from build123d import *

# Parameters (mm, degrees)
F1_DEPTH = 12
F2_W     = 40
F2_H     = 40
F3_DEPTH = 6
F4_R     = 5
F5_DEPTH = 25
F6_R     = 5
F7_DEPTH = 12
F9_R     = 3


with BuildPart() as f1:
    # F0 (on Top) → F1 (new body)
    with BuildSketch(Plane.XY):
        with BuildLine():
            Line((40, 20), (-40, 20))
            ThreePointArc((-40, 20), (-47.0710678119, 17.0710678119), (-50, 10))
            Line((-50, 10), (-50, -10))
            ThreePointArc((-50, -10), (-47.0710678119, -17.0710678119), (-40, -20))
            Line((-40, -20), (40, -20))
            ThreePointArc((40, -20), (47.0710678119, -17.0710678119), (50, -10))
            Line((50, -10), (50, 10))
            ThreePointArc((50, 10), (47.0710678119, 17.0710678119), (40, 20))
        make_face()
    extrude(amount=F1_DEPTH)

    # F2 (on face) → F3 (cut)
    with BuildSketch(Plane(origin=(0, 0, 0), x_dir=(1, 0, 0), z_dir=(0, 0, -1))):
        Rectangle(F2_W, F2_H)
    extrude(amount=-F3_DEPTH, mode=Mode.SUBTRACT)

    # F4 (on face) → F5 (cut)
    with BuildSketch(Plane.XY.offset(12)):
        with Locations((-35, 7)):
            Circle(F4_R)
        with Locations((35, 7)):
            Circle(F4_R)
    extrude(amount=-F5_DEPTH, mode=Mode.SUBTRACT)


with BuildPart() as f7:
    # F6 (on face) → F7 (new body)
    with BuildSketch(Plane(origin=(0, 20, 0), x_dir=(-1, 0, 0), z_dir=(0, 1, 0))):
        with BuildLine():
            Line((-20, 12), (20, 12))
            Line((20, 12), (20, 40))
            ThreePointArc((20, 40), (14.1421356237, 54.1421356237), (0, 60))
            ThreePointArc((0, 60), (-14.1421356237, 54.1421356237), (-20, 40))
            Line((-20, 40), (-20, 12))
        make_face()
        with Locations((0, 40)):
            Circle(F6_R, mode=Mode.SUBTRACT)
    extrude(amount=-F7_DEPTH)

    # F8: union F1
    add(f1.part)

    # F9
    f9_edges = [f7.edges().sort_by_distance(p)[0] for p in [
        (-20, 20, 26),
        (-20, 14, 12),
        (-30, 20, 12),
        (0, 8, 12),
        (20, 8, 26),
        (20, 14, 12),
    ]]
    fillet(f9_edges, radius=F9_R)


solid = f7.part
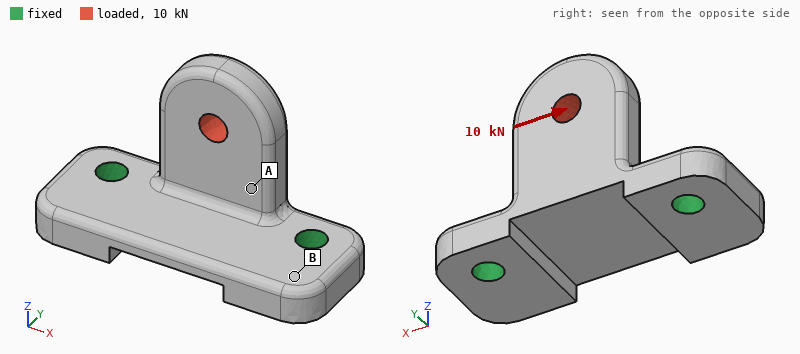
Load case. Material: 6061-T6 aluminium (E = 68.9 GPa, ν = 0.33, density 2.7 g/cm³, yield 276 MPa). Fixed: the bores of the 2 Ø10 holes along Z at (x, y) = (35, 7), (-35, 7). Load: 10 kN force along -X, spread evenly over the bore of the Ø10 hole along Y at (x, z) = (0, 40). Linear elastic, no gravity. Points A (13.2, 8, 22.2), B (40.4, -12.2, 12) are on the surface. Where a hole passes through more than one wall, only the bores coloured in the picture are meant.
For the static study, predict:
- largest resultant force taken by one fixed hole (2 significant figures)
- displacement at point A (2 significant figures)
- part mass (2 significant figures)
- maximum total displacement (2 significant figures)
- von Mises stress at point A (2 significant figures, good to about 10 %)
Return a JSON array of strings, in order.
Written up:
["8.6 kN", "0.053 mm", "150 g", "0.17 mm", "72 MPa"]
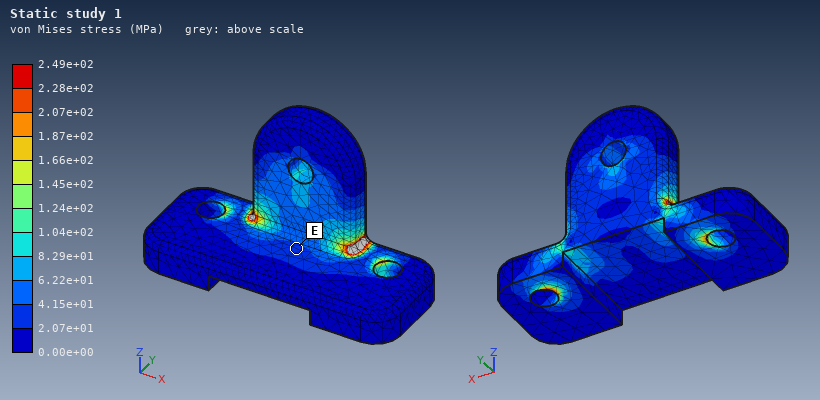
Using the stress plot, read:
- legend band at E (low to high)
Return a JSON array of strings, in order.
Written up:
["2.07e+01 to 4.15e+01 MPa"]
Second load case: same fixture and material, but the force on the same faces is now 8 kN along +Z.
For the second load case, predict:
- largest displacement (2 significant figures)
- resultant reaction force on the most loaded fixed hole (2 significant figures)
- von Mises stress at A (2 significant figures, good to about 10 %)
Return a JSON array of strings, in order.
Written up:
["0.11 mm", "4.9 kN", "28 MPa"]
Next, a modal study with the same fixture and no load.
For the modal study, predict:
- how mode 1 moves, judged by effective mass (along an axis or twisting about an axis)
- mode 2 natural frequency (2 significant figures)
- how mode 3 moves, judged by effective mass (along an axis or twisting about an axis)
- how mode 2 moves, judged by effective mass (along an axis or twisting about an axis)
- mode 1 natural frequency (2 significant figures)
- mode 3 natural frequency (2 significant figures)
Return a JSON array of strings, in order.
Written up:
["along Y", "6900 Hz", "along Z", "along X", "2600 Hz", "9300 Hz"]
